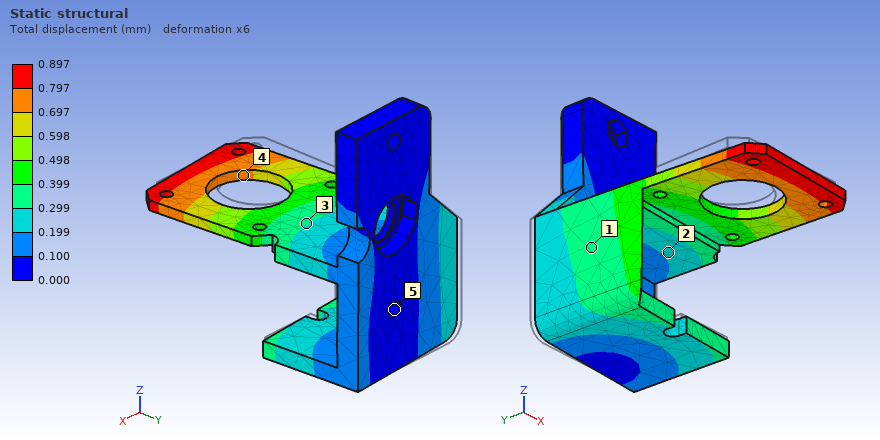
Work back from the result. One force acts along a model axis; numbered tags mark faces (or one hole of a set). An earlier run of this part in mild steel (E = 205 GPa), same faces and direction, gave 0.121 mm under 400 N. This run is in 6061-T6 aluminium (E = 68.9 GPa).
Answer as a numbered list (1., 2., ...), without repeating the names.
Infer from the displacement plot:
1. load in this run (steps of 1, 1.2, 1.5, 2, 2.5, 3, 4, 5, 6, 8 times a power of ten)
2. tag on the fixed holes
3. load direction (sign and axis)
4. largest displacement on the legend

1. 1 kN
2. 5
3. +X
4. 0.897 mm
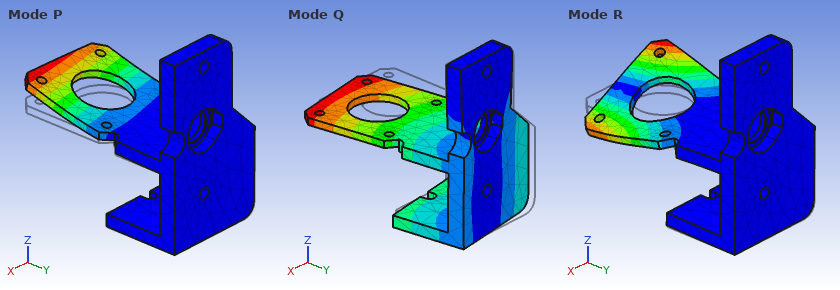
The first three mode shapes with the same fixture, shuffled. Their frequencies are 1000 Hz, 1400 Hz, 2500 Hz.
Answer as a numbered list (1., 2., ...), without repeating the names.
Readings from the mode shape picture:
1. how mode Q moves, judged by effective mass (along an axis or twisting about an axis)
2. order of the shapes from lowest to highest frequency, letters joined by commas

1. along X
2. P, Q, R
